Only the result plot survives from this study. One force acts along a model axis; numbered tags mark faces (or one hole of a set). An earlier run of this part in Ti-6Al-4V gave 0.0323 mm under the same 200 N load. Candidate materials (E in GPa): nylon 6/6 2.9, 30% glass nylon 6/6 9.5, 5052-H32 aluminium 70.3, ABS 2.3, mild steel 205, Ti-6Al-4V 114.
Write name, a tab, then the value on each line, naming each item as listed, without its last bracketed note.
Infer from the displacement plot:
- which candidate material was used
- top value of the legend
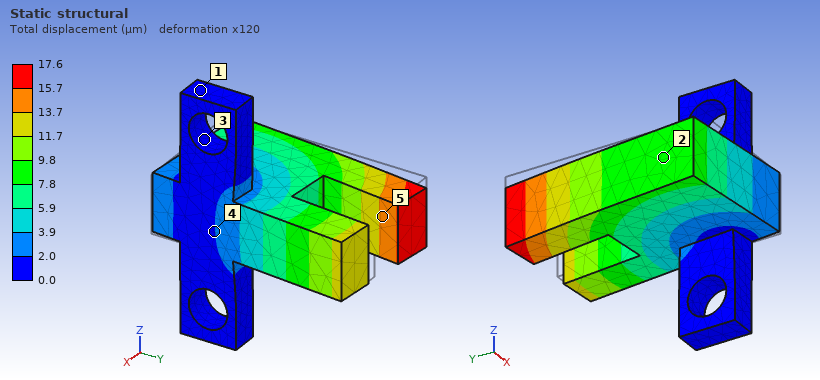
which candidate material was used	mild steel
top value of the legend	17.6 µm
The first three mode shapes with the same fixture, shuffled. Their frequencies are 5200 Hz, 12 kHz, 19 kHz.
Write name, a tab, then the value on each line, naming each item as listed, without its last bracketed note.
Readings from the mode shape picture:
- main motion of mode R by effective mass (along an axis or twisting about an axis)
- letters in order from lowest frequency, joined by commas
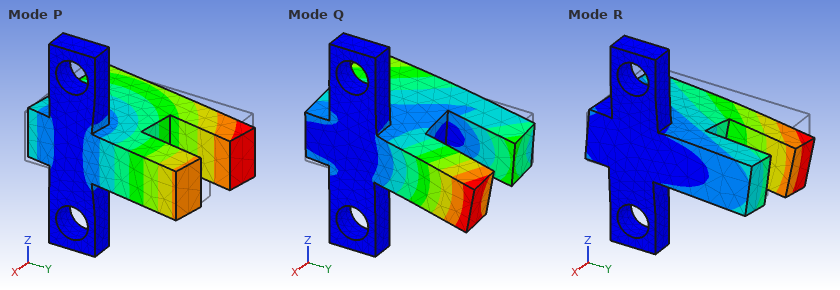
main motion of mode R by effective mass	along Z
letters in order from lowest frequency, joined by commas	P, R, Q
